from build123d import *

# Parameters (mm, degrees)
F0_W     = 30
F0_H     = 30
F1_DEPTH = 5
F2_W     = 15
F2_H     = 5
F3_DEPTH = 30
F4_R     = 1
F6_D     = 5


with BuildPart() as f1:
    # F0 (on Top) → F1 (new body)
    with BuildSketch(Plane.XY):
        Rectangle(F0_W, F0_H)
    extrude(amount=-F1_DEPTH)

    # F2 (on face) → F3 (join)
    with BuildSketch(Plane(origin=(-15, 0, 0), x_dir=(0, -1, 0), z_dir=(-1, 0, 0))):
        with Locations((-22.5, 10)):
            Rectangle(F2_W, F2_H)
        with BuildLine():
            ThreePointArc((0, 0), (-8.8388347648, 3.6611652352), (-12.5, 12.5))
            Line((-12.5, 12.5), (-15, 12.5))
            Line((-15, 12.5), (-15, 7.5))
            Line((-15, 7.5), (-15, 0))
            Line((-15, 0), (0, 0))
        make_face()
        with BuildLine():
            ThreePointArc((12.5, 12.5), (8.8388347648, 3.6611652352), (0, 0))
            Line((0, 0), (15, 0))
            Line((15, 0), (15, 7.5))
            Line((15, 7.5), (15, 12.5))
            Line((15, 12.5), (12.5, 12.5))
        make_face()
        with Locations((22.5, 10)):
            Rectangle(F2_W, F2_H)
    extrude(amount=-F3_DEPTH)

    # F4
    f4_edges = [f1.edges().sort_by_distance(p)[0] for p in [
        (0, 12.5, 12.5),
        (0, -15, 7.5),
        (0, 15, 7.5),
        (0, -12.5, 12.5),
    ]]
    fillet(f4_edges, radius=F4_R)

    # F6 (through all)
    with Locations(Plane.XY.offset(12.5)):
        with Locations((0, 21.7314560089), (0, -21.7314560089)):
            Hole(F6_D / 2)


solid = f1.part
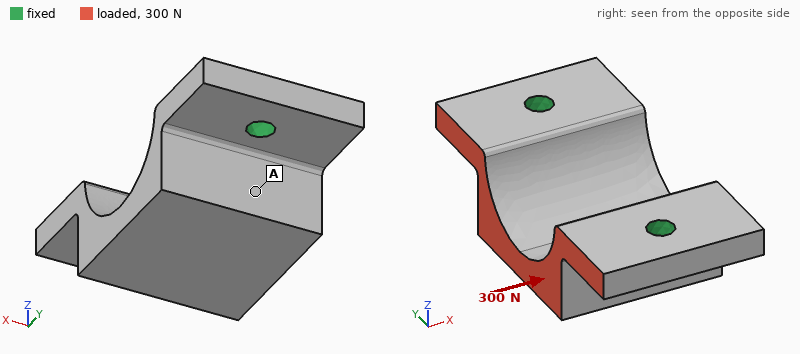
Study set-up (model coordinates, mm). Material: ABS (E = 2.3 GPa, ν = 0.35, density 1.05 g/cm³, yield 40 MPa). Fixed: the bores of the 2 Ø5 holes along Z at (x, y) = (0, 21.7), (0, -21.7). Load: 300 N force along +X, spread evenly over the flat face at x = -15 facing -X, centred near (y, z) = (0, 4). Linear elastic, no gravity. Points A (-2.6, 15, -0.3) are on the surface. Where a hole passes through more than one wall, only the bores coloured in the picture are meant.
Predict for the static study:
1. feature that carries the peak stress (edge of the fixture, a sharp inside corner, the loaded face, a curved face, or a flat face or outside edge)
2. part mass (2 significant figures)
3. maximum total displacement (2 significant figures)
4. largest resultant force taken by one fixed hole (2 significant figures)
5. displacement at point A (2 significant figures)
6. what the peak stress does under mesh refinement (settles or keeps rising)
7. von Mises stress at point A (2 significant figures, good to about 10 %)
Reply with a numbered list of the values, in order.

1. edge of the fixture
2. 13 g
3. 0.20 mm
4. 150 N
5. 0.11 mm
6. keeps rising
7. 1.8 MPa
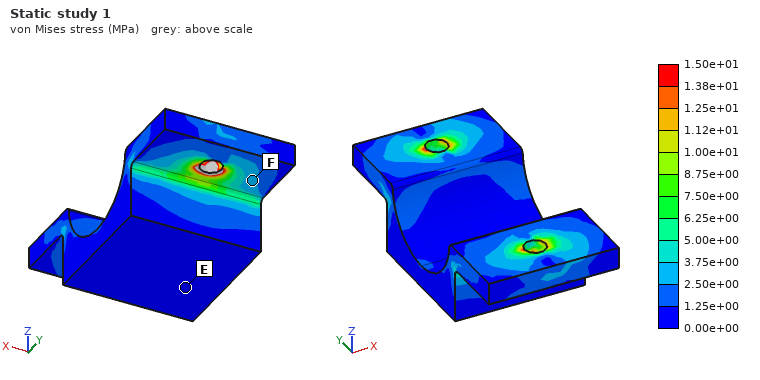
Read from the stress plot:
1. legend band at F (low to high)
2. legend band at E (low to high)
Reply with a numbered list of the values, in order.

1. 2.50e+00 to 3.75e+00 MPa
2. 0.00e+00 to 1.25e+00 MPa
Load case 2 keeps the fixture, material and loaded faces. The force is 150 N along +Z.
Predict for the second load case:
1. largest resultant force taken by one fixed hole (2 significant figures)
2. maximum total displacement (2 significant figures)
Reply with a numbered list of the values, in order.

1. 80 N
2. 0.19 mm
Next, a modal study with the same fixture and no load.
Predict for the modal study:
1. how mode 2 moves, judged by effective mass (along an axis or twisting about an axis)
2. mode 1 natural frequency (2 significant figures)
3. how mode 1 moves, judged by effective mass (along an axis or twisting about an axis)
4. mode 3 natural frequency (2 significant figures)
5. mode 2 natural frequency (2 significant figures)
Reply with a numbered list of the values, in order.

1. along Z
2. 1800 Hz
3. along X
4. 4600 Hz
5. 4400 Hz
